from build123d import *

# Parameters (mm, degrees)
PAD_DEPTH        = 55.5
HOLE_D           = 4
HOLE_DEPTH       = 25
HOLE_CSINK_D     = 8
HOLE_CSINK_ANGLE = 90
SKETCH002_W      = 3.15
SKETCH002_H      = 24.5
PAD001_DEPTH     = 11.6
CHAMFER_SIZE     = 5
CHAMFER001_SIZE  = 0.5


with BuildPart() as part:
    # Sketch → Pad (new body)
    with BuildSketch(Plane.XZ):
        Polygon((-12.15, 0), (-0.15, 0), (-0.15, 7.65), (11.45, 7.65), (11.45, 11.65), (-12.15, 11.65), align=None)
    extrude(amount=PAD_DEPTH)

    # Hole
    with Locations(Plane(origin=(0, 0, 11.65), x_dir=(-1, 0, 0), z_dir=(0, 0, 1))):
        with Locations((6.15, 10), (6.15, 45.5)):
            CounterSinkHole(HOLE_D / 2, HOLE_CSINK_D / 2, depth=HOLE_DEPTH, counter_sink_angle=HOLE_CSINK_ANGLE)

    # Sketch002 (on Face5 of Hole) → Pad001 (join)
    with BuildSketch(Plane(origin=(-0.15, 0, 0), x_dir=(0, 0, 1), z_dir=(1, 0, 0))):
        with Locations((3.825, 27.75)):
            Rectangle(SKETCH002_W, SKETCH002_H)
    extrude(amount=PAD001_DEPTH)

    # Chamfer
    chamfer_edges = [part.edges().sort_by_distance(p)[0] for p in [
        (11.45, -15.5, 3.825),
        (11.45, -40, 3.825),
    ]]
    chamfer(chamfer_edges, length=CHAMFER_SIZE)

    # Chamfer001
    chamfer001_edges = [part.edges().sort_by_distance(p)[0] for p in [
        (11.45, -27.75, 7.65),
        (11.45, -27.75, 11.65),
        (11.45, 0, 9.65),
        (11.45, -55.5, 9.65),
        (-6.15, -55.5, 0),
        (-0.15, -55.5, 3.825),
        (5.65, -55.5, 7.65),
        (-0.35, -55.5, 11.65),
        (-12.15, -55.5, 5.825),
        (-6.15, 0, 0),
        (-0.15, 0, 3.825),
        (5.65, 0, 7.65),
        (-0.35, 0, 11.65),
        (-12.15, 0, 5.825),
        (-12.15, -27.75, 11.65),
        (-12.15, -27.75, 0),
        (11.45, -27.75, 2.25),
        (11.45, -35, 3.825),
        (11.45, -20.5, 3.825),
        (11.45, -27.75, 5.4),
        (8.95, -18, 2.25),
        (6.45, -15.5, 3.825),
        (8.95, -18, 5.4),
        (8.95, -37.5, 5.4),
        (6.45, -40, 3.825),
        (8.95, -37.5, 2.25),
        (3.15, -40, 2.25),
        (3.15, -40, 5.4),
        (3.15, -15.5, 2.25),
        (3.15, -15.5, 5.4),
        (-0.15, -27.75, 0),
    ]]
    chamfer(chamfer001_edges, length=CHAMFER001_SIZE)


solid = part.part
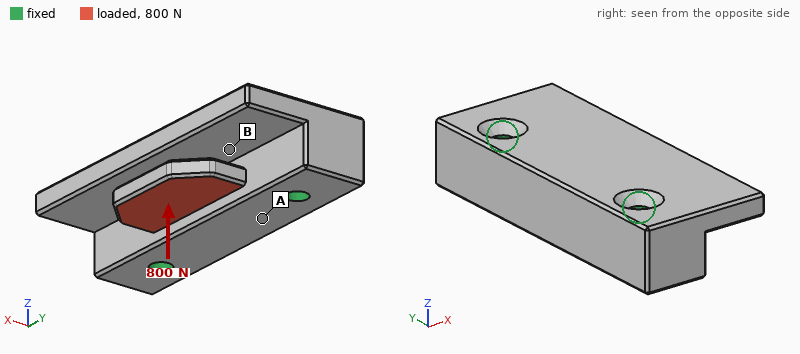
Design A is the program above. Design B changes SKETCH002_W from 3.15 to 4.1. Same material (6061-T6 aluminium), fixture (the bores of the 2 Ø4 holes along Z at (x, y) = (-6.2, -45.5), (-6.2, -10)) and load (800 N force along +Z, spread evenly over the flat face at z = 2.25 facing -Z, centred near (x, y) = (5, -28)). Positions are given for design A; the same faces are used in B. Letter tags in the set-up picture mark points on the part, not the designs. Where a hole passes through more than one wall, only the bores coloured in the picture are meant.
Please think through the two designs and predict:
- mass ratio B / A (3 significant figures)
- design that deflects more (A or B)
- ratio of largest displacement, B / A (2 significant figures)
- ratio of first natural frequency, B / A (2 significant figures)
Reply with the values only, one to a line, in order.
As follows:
1.02
A
0.63
1.0
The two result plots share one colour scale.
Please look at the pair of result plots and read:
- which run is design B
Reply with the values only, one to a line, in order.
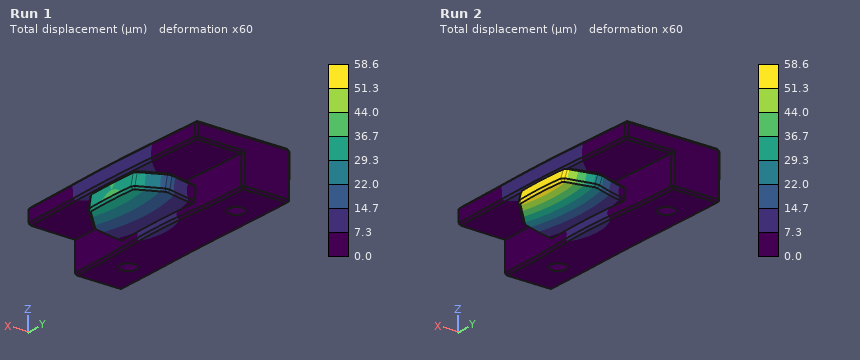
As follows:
Run 1
